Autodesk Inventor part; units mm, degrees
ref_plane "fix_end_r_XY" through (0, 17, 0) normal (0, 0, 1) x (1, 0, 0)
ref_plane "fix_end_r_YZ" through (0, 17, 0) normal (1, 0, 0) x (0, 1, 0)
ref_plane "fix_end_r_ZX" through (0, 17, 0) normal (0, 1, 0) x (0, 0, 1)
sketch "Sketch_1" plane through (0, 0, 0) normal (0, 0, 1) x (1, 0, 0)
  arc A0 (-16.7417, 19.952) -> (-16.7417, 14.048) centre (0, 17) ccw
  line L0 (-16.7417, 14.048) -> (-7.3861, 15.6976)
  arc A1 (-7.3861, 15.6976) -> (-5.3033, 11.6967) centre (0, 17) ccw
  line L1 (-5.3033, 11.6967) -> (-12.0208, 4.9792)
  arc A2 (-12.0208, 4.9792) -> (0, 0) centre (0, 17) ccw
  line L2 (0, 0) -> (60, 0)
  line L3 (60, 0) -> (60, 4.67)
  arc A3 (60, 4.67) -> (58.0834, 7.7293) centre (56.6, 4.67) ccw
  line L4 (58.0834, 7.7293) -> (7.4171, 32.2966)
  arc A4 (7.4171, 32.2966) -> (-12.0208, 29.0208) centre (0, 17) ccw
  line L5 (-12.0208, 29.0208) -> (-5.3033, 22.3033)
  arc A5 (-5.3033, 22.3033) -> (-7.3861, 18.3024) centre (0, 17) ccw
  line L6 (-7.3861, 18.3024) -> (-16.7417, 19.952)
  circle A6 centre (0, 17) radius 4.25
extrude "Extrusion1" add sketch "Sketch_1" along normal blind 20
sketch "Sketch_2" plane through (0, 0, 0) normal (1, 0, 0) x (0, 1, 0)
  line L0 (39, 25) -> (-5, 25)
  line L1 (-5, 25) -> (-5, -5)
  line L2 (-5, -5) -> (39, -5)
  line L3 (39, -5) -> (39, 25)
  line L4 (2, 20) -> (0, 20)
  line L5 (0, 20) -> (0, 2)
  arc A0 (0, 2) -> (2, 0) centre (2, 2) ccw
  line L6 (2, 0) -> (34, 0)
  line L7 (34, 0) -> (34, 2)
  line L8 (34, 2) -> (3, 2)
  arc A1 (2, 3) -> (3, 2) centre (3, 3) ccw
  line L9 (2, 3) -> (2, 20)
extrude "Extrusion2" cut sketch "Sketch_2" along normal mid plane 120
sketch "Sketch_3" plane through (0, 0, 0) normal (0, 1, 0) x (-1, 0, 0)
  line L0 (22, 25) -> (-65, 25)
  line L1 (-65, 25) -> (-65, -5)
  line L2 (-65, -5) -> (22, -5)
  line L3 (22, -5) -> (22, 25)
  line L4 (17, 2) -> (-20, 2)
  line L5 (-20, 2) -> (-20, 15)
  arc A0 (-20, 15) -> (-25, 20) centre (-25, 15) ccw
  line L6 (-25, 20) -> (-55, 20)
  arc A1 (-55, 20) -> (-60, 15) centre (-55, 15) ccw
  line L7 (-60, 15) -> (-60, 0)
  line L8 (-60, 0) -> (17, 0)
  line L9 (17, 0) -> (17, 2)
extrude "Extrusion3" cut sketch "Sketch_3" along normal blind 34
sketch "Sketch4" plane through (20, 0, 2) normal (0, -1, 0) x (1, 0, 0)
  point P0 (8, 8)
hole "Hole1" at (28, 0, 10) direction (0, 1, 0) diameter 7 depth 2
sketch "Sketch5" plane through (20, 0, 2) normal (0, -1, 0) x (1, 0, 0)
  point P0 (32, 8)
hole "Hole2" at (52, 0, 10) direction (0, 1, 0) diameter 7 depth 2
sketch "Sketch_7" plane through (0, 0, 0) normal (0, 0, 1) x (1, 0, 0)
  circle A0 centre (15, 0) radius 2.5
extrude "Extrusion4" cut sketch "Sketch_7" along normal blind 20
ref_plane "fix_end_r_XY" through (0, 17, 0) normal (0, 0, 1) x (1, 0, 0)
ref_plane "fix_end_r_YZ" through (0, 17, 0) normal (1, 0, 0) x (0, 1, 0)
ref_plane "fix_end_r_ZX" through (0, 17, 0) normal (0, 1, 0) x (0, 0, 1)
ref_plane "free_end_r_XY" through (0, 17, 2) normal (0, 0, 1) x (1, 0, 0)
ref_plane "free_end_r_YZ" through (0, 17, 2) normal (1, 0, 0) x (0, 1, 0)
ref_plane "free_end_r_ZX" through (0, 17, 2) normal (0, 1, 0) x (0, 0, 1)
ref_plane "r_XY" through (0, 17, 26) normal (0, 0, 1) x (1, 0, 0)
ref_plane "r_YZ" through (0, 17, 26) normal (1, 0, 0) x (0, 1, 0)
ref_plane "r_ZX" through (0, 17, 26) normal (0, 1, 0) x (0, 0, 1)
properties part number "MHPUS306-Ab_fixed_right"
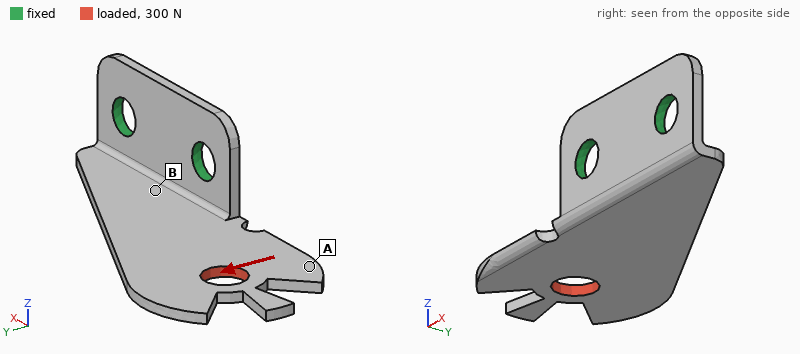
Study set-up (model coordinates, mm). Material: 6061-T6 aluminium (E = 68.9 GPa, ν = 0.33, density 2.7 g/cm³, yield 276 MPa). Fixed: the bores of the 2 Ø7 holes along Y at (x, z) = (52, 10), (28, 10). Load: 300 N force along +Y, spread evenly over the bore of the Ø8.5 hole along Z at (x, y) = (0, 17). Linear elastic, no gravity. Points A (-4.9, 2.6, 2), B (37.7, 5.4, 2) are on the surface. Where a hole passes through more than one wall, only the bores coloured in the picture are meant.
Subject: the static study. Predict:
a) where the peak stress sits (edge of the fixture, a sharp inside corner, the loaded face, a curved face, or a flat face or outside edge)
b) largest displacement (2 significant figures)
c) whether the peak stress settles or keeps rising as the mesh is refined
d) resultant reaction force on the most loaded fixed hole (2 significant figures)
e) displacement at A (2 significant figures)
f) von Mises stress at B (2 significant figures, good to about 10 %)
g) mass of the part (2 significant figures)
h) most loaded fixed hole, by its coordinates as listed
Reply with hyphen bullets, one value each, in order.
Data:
- edge of the fixture
- 0.52 mm
- keeps rising
- 620 N
- 0.24 mm
- 55 MPa
- 12 g
- (28, 10)
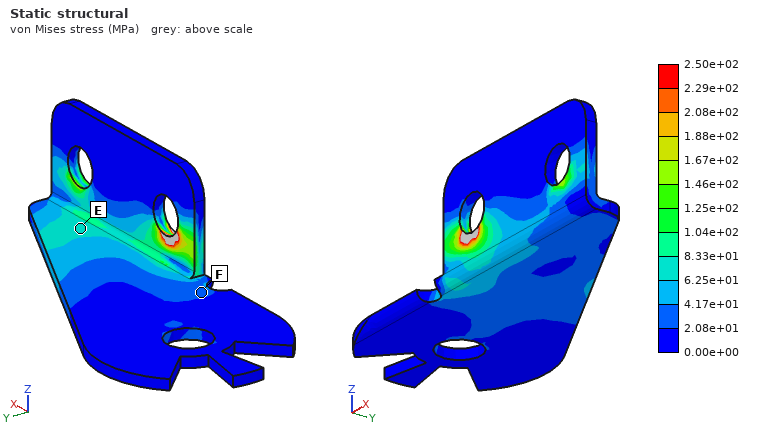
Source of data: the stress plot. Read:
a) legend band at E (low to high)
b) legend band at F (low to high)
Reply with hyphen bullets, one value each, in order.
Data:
- 6.25e+01 to 8.33e+01 MPa
- 2.08e+01 to 4.17e+01 MPa
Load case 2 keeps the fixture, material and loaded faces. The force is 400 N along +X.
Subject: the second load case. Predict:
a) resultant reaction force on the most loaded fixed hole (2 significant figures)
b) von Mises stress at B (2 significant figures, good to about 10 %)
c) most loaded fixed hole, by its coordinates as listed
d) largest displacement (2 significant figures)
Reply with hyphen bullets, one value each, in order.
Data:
- 350 N
- 33 MPa
- (52, 10)
- 0.20 mm
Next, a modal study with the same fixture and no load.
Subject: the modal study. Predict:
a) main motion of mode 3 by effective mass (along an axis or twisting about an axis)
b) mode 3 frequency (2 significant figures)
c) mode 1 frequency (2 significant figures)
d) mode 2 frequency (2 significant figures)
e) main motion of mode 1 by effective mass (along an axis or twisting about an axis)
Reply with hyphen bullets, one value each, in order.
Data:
- along Y
- 3000 Hz
- 770 Hz
- 2000 Hz
- along Z
